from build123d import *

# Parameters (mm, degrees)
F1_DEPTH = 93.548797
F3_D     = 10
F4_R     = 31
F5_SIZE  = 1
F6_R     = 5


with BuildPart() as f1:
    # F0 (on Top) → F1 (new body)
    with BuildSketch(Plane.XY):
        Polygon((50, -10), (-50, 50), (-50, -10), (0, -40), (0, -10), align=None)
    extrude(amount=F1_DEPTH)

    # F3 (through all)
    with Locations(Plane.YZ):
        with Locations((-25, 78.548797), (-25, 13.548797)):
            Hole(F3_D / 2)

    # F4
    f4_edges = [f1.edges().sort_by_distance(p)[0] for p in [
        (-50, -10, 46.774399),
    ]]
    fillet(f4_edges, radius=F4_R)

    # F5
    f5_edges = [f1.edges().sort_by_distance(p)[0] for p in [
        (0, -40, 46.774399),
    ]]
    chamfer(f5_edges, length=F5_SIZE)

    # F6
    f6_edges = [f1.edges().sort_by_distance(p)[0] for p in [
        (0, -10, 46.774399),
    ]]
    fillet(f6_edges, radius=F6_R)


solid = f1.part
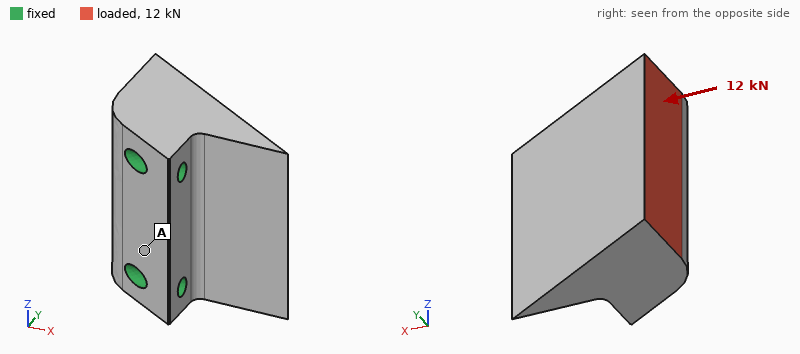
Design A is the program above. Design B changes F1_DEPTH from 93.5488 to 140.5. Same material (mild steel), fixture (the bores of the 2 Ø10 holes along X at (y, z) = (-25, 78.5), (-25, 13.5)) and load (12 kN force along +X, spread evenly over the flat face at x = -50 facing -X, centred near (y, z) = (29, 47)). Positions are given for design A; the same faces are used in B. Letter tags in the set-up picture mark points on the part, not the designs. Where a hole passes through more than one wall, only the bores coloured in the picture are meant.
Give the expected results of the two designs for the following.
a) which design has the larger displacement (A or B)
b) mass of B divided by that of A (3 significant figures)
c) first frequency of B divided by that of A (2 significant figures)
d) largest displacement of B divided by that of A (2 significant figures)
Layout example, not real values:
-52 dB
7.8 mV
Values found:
B
1.51
0.79
1.1
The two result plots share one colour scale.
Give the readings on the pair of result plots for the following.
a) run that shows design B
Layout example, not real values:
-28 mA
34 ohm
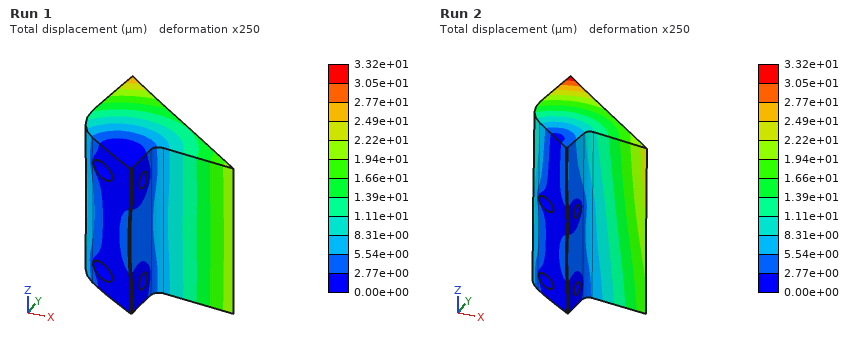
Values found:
Run 2
